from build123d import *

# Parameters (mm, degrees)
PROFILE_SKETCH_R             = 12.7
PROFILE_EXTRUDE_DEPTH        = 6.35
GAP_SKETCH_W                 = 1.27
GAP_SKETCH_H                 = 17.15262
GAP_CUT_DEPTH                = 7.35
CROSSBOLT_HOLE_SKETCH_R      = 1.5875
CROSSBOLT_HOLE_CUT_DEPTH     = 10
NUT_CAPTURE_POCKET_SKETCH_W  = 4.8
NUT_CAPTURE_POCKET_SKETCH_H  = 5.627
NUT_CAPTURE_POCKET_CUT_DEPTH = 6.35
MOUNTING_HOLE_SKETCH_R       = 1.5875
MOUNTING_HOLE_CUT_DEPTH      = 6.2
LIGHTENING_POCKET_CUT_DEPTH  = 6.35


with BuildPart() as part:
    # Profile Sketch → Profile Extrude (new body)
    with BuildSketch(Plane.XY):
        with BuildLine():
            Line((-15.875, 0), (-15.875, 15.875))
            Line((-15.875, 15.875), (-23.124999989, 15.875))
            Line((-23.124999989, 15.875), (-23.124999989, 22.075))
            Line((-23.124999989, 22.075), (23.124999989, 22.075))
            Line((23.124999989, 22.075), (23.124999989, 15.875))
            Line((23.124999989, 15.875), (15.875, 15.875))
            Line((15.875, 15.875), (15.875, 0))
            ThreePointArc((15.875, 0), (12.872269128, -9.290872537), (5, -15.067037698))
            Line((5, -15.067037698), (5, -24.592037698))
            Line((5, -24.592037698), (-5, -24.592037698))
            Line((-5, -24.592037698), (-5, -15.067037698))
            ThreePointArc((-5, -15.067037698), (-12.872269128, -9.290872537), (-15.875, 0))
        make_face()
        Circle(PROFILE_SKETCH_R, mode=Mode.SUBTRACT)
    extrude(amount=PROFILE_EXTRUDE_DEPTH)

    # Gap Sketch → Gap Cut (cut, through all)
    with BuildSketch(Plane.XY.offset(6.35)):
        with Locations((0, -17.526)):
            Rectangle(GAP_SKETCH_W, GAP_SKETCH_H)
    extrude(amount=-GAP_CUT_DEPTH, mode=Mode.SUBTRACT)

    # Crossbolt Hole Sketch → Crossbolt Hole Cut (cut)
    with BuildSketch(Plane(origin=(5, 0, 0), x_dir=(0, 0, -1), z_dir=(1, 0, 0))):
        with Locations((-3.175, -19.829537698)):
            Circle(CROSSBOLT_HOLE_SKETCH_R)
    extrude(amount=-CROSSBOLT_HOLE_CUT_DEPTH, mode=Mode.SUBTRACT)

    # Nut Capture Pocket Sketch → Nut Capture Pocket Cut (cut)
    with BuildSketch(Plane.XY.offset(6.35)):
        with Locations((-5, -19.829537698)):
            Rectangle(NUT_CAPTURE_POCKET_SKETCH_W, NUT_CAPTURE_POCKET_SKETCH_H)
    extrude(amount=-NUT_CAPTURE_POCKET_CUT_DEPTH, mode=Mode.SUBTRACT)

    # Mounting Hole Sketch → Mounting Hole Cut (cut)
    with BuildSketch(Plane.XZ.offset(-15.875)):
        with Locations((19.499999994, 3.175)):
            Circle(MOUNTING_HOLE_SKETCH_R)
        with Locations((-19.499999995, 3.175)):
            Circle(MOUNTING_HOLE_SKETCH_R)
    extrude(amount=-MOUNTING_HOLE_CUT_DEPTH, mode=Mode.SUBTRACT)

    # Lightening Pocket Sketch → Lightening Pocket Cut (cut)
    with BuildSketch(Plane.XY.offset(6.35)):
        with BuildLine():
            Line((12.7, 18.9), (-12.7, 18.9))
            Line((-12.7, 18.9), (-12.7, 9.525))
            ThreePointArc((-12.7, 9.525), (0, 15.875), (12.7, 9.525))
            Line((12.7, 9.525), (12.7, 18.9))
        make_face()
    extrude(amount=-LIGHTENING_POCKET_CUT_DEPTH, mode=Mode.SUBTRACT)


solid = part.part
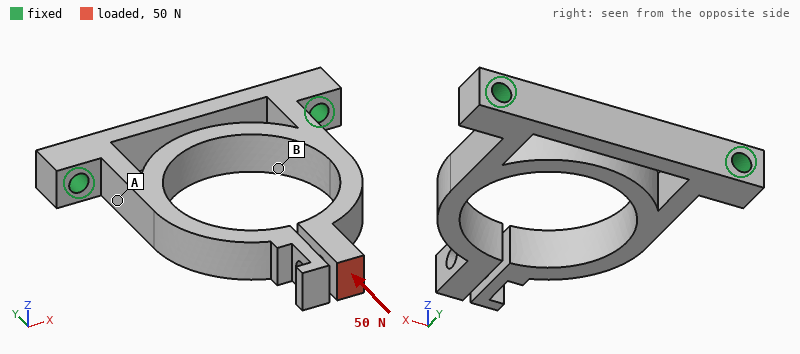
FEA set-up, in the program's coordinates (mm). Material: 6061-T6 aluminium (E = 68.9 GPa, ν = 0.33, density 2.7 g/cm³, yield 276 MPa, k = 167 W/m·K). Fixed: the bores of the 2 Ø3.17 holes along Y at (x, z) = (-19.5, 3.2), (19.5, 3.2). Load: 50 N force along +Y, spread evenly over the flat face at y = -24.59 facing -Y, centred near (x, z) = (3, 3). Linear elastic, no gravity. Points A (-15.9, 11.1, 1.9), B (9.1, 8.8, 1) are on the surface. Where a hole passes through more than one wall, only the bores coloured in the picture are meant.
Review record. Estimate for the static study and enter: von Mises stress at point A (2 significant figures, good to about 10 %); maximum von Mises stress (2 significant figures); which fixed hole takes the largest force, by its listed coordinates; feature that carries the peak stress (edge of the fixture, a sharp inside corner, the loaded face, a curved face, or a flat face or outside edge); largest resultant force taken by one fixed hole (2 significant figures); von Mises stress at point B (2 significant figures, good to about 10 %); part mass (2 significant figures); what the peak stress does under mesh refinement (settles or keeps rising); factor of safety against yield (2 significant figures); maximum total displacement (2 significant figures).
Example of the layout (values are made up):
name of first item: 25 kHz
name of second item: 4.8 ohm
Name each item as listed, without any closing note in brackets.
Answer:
von Mises stress at point A: 8.4 MPa
maximum von Mises stress: 60 MPa
which fixed hole takes the largest force, by its listed coordinates: (19.5, 3.2)
feature that carries the peak stress: a curved face
largest resultant force taken by one fixed hole: 35 N
von Mises stress at point B: 23 MPa
part mass: 10 g
what the peak stress does under mesh refinement: settles
factor of safety against yield: 4.6
maximum total displacement: 0.28 mm
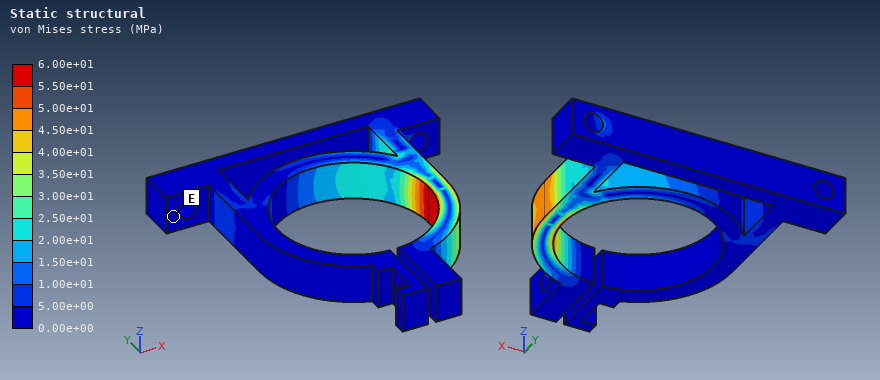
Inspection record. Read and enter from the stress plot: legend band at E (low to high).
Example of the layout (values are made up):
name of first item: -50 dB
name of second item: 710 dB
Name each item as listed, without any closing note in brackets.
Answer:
legend band at E: 0.00e+00 to 5.00e+00 MPa
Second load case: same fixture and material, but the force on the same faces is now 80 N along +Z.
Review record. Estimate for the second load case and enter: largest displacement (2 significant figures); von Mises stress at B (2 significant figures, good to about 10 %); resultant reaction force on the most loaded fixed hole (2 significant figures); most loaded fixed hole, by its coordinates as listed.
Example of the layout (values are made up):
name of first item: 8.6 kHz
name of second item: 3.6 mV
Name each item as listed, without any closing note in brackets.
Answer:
largest displacement: 0.64 mm
von Mises stress at B: 32 MPa
resultant reaction force on the most loaded fixed hole: 60 N
most loaded fixed hole, by its coordinates as listed: (19.5, 3.2)
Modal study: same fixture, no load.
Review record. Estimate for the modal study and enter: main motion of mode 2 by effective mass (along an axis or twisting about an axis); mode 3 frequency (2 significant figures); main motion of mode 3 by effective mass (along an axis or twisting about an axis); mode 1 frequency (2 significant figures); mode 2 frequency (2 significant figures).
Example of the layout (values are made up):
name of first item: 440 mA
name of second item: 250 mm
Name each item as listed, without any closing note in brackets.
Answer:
main motion of mode 2 by effective mass: along X
mode 3 frequency: 2000 Hz
main motion of mode 3 by effective mass: along Z
mode 1 frequency: 1500 Hz
mode 2 frequency: 1800 Hz
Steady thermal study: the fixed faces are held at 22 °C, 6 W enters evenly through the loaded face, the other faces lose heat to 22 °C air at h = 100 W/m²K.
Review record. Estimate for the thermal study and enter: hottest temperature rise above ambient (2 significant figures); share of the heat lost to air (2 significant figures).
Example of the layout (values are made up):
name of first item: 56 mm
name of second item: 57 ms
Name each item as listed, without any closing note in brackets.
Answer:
hottest temperature rise above ambient: 55 K
share of the heat lost to air: 49 %
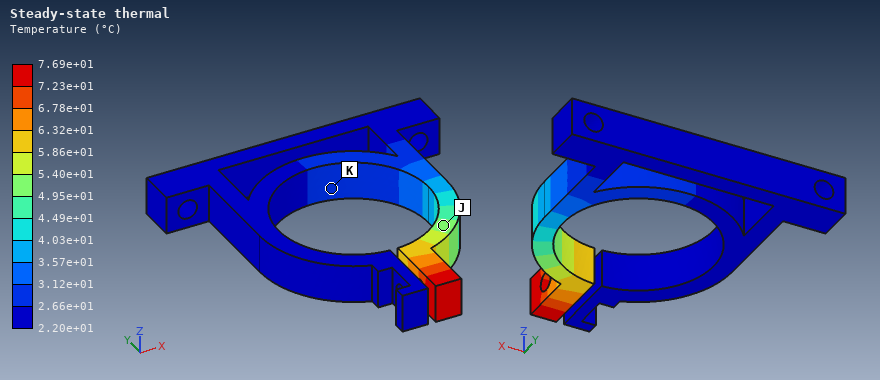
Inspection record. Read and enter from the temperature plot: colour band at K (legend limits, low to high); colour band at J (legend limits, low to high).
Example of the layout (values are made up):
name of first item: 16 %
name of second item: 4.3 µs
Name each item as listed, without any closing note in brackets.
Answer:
colour band at K: 2.66e+01 to 3.12e+01 °C
colour band at J: 4.95e+01 to 5.40e+01 °C
